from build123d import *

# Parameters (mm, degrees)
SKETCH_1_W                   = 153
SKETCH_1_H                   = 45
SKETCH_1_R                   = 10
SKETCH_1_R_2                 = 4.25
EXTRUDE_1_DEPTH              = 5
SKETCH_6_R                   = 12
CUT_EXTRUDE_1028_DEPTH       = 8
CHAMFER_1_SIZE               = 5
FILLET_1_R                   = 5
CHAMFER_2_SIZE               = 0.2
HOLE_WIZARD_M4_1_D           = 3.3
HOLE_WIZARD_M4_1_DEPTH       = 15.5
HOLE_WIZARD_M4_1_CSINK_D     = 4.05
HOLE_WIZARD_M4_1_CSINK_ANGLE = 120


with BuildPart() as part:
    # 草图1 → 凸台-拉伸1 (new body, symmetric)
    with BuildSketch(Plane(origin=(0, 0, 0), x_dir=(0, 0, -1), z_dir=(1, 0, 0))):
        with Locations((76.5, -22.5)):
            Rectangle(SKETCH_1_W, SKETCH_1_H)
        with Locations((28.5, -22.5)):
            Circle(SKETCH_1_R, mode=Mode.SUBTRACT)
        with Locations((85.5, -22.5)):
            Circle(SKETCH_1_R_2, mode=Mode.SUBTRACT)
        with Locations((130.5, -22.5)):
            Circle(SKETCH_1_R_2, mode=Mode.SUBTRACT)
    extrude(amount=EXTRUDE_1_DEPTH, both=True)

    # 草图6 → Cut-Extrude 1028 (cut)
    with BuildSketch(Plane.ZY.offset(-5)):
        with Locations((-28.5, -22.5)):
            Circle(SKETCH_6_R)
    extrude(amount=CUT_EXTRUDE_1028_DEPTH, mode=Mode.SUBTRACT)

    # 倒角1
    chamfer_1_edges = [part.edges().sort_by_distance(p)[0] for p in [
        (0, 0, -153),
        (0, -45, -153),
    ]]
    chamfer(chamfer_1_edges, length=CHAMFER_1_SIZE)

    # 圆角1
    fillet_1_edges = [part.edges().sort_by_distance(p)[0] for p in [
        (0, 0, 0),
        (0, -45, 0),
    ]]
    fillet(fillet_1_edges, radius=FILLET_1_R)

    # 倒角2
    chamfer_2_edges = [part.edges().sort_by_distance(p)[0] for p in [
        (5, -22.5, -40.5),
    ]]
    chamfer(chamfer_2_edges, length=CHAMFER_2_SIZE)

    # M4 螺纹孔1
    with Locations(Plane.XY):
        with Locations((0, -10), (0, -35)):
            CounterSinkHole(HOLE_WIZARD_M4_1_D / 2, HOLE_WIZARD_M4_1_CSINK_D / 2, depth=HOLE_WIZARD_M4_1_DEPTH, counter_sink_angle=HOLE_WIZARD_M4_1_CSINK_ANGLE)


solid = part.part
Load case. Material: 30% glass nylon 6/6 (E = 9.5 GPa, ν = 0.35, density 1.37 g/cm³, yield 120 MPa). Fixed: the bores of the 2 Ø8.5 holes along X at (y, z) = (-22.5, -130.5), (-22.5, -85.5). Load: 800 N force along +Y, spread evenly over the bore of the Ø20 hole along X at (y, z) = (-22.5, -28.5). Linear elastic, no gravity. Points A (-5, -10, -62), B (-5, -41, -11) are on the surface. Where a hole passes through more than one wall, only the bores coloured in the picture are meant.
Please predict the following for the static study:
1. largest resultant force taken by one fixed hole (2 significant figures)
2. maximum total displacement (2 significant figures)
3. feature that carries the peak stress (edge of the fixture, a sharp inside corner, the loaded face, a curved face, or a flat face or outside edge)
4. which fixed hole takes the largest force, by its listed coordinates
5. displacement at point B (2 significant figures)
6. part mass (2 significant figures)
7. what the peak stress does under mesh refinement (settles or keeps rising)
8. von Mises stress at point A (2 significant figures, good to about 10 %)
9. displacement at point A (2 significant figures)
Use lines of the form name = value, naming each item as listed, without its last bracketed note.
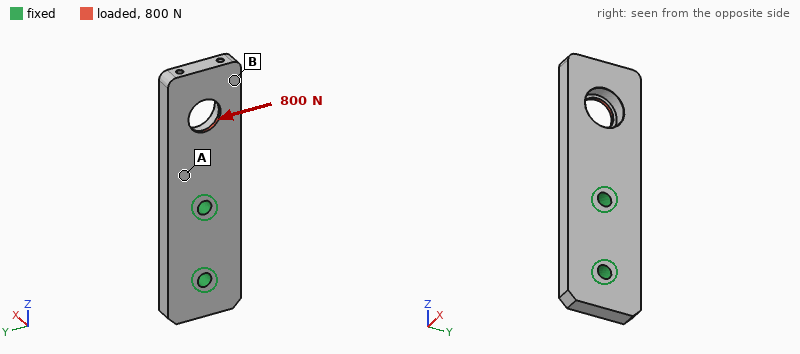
largest resultant force taken by one fixed hole = 1.5 kN
maximum total displacement = 0.34 mm
feature that carries the peak stress = edge of the fixture
which fixed hole takes the largest force, by its listed coordinates = (-22.5, -85.5)
displacement at point B = 0.30 mm
part mass = 86 g
what the peak stress does under mesh refinement = keeps rising
von Mises stress at point A = 7.8 MPa
displacement at point A = 0.074 mm
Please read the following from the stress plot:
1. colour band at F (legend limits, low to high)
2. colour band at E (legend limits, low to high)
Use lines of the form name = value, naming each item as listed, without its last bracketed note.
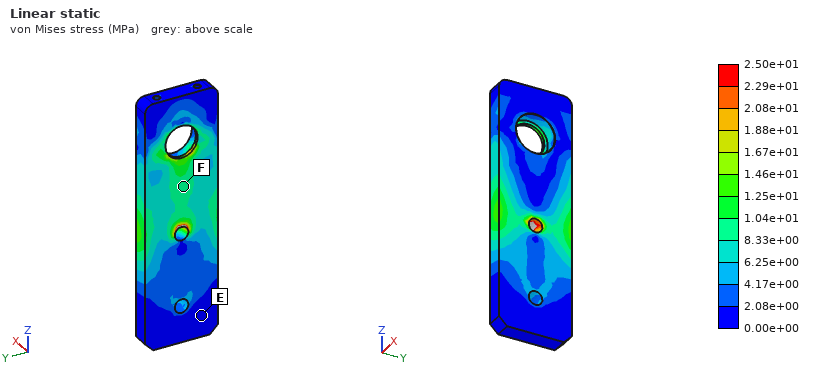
colour band at F = 8.33e+00 to 1.04e+01 MPa
colour band at E = 0.00e+00 to 2.08e+00 MPa
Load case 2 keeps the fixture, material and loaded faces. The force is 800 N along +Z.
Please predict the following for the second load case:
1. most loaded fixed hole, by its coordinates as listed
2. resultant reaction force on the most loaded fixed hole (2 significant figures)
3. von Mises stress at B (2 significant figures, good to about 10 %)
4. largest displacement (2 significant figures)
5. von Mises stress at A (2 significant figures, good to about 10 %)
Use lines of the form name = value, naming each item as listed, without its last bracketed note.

most loaded fixed hole, by its coordinates as listed = (-22.5, -85.5)
resultant reaction force on the most loaded fixed hole = 660 N
von Mises stress at B = 1.6 MPa
largest displacement = 0.31 mm
von Mises stress at A = 5.9 MPa
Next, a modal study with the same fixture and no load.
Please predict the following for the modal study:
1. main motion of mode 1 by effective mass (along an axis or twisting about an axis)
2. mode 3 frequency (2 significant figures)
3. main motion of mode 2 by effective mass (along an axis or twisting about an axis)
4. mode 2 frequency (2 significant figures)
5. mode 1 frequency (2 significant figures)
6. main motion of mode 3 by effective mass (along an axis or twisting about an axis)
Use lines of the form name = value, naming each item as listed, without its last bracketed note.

main motion of mode 1 by effective mass = along X
mode 3 frequency = 1900 Hz
main motion of mode 2 by effective mass = along Y
mode 2 frequency = 1700 Hz
mode 1 frequency = 620 Hz
main motion of mode 3 by effective mass = twisting about Z
